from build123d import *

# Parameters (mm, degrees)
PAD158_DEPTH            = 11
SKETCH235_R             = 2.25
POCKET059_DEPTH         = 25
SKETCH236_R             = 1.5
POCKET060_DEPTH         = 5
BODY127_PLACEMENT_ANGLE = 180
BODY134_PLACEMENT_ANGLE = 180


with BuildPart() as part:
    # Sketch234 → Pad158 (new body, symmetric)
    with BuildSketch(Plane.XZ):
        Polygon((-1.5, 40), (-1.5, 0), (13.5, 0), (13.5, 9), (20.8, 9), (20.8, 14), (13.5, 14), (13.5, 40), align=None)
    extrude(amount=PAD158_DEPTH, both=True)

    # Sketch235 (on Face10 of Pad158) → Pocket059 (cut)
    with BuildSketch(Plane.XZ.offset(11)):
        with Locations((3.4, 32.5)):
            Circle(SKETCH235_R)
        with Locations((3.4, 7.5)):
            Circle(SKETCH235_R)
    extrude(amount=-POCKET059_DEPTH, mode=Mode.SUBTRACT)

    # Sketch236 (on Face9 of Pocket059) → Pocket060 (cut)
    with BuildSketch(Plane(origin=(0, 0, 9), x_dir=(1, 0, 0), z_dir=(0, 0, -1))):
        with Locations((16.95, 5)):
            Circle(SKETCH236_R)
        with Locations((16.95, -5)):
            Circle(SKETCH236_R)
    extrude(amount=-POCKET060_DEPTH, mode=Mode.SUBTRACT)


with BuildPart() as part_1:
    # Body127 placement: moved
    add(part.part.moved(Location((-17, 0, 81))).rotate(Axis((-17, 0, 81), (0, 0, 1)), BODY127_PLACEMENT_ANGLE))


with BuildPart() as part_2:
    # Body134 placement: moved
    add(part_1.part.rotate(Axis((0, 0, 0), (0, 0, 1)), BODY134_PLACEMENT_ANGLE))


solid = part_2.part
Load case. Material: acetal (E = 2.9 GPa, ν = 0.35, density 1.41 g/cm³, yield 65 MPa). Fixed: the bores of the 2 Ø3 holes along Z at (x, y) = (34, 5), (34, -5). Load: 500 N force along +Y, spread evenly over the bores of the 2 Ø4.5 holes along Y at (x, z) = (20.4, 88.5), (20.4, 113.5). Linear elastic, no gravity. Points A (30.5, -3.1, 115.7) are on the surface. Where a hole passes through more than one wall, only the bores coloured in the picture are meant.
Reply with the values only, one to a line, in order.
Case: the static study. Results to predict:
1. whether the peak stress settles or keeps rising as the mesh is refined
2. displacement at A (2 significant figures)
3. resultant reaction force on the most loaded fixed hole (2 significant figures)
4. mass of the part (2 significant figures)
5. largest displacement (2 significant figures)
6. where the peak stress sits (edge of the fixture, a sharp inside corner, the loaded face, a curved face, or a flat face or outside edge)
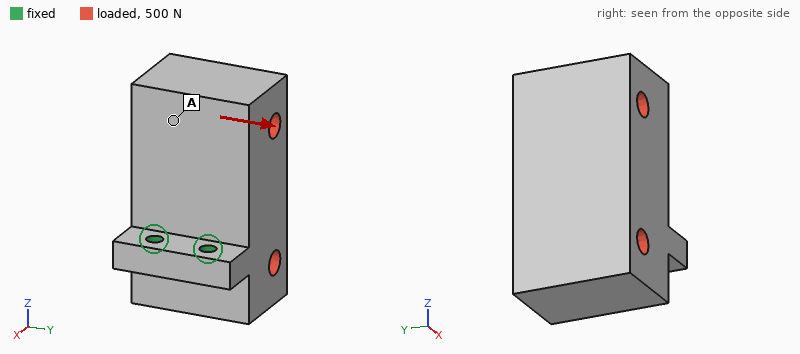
keeps rising
0.23 mm
660 N
19 g
0.37 mm
edge of the fixture
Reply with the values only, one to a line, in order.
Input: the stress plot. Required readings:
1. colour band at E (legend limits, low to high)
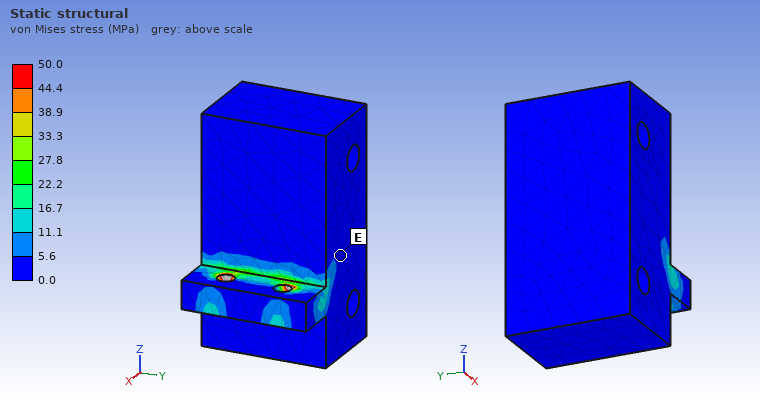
0.0 to 5.6 MPa
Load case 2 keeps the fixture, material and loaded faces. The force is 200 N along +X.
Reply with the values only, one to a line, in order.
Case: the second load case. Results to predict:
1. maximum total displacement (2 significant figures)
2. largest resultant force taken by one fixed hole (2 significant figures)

0.46 mm
100 N
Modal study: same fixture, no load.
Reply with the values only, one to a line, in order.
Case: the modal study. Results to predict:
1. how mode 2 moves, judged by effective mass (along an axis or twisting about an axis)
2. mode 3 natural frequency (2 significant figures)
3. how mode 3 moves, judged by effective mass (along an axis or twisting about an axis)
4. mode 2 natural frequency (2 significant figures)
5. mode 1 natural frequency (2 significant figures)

along Y
3400 Hz
along Y
1700 Hz
780 Hz
